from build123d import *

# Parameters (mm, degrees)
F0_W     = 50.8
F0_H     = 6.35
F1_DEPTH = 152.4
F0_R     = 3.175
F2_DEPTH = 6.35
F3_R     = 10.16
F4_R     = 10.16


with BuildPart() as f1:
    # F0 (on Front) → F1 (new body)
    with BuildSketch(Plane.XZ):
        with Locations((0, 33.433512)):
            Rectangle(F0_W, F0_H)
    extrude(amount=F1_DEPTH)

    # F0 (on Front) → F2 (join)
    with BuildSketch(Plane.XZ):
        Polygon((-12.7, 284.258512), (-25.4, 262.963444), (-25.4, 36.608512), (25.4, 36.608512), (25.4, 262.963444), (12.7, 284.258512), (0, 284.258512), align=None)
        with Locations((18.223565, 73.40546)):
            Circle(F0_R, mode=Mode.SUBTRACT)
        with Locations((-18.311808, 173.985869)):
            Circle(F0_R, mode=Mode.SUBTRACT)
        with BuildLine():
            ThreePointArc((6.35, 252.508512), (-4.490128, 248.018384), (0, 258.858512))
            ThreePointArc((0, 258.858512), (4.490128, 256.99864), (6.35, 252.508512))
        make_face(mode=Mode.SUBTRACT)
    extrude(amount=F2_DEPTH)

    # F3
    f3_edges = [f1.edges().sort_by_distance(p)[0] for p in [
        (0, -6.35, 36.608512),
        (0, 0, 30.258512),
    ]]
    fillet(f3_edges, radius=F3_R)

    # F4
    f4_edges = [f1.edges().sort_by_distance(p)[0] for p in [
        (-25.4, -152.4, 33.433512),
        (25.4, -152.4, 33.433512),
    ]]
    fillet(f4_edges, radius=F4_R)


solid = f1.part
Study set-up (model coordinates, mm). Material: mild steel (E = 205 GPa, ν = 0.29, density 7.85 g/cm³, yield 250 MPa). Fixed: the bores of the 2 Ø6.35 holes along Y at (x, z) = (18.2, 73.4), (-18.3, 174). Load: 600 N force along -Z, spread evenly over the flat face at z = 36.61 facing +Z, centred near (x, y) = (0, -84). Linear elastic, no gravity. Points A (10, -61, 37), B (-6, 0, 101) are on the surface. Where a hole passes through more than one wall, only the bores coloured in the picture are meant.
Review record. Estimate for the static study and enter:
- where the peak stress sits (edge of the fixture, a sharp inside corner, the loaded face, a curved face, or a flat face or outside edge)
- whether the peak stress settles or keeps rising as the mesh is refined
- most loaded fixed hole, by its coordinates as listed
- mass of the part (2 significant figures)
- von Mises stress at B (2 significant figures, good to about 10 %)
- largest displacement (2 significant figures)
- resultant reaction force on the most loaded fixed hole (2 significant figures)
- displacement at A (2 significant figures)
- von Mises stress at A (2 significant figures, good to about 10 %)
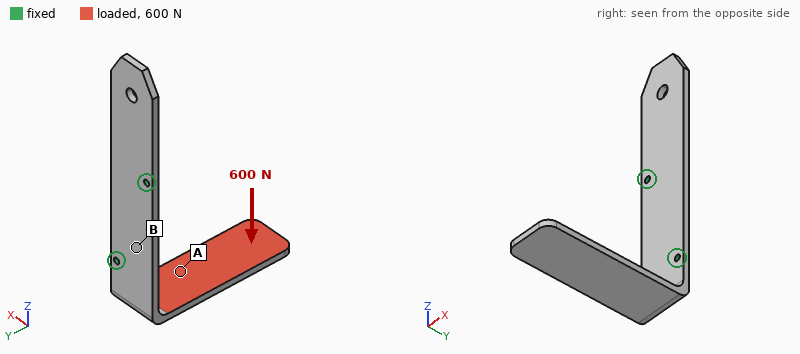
edge of the fixture
keeps rising
(18.2, 73.4)
990 g
22 MPa
2.3 mm
470 N
0.71 mm
53 MPa
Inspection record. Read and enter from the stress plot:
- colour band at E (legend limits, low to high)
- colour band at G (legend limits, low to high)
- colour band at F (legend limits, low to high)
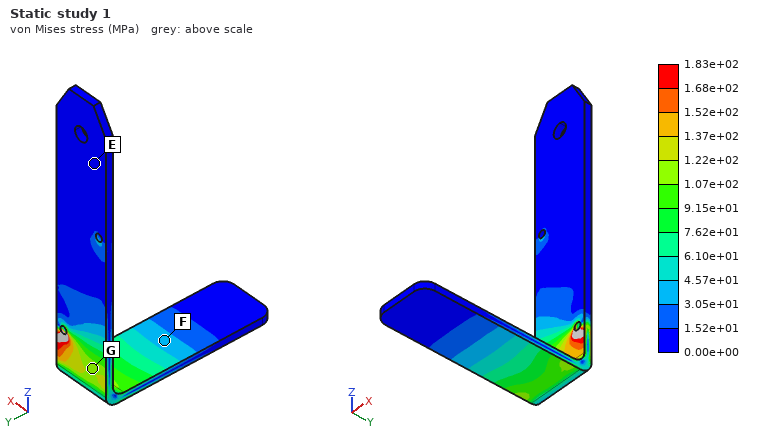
0.00e+00 to 1.52e+01 MPa
1.07e+02 to 1.22e+02 MPa
3.05e+01 to 4.57e+01 MPa
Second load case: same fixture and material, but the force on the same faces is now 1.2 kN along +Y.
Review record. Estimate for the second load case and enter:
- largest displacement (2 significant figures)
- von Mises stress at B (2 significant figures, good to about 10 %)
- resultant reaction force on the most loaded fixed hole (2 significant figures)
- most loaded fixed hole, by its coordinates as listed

0.68 mm
24 MPa
1.3 kN
(18.2, 73.4)
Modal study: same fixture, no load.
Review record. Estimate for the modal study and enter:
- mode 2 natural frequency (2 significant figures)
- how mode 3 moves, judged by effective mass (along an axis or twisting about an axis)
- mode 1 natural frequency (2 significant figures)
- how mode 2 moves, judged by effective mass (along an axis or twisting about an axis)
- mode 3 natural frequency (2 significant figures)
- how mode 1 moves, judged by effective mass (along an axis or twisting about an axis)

260 Hz
along Y
170 Hz
along X
430 Hz
along Z
